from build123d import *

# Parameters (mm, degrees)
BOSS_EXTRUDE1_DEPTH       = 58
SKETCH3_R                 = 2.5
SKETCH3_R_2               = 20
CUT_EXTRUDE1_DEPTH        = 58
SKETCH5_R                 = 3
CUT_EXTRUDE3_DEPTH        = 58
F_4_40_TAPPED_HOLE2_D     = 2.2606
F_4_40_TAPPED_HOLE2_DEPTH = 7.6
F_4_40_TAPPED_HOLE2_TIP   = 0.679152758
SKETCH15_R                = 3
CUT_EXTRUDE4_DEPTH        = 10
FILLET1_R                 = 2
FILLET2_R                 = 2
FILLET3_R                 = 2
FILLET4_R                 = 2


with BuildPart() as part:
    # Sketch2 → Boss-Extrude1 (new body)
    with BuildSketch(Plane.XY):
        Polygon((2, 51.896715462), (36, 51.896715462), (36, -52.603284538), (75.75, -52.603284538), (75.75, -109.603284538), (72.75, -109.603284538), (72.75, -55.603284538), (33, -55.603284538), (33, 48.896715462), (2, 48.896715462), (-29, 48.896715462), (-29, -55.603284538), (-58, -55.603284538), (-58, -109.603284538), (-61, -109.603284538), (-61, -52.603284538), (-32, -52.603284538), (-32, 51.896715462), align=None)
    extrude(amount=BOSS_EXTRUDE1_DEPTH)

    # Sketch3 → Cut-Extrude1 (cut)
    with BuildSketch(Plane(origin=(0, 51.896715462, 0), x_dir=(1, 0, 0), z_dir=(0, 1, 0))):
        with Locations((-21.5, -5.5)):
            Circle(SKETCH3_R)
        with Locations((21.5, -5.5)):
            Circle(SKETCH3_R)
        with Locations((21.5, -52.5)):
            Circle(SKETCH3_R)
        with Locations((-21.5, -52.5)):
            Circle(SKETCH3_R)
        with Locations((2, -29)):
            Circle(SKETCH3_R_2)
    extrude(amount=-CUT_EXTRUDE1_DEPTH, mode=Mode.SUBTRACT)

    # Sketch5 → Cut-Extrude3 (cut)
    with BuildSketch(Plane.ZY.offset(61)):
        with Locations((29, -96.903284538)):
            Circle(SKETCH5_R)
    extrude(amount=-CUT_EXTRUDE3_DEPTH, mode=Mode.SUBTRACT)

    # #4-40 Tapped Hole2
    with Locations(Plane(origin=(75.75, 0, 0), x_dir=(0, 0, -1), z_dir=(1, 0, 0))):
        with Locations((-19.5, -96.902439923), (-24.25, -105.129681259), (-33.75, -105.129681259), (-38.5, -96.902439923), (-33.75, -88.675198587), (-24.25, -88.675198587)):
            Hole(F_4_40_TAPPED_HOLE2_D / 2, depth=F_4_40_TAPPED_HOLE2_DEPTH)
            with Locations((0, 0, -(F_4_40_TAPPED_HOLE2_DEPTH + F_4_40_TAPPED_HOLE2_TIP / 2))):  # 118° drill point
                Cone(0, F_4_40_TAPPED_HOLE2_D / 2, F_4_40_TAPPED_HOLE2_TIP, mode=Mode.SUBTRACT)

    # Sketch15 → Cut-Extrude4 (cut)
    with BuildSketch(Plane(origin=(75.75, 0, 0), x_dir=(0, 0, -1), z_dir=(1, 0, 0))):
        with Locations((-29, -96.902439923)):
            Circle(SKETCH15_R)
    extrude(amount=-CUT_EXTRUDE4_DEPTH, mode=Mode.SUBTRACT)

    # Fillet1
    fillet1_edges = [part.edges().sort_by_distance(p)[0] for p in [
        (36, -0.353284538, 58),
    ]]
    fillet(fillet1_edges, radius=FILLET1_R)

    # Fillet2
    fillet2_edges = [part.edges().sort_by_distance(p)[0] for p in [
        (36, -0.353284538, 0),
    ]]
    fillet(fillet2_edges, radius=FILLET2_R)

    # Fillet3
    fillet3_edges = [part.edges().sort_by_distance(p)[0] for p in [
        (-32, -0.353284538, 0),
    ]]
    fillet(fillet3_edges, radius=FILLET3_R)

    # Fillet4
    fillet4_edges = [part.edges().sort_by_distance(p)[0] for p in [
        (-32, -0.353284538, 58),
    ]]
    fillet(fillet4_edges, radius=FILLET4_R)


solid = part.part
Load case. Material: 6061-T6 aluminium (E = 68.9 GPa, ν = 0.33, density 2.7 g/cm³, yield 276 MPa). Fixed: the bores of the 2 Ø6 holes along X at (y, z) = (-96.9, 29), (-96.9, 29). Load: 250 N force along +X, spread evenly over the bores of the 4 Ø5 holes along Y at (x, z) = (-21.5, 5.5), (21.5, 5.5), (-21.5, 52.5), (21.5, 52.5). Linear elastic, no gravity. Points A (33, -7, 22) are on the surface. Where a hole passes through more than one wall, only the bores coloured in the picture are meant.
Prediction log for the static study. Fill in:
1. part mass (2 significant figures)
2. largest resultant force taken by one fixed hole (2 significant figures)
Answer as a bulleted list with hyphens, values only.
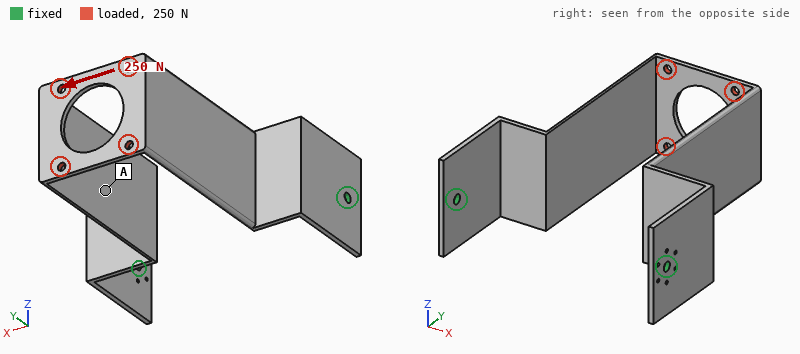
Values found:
- 200 g
- 260 N
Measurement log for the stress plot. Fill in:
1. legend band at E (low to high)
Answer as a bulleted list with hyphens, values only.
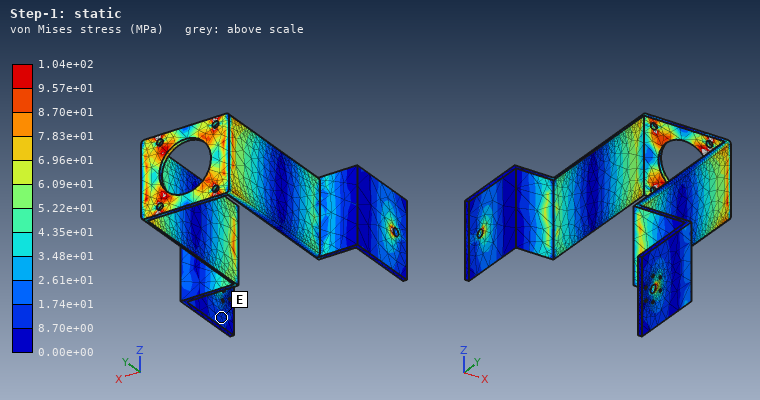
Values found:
- 8.70e+00 to 1.74e+01 MPa
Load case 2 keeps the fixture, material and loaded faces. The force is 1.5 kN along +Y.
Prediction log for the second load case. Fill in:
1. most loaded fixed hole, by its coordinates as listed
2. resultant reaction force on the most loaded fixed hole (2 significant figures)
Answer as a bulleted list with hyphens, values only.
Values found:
- (-96.9, 29)
- 850 N
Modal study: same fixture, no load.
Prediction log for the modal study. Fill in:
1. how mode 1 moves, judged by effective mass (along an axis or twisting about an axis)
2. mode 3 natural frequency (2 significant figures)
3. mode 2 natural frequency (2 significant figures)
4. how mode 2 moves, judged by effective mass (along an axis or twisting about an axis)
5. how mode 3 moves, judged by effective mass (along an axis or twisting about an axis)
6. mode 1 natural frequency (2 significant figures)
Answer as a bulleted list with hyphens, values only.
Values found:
- along X
- 330 Hz
- 210 Hz
- along Z
- along Y
- 190 Hz
